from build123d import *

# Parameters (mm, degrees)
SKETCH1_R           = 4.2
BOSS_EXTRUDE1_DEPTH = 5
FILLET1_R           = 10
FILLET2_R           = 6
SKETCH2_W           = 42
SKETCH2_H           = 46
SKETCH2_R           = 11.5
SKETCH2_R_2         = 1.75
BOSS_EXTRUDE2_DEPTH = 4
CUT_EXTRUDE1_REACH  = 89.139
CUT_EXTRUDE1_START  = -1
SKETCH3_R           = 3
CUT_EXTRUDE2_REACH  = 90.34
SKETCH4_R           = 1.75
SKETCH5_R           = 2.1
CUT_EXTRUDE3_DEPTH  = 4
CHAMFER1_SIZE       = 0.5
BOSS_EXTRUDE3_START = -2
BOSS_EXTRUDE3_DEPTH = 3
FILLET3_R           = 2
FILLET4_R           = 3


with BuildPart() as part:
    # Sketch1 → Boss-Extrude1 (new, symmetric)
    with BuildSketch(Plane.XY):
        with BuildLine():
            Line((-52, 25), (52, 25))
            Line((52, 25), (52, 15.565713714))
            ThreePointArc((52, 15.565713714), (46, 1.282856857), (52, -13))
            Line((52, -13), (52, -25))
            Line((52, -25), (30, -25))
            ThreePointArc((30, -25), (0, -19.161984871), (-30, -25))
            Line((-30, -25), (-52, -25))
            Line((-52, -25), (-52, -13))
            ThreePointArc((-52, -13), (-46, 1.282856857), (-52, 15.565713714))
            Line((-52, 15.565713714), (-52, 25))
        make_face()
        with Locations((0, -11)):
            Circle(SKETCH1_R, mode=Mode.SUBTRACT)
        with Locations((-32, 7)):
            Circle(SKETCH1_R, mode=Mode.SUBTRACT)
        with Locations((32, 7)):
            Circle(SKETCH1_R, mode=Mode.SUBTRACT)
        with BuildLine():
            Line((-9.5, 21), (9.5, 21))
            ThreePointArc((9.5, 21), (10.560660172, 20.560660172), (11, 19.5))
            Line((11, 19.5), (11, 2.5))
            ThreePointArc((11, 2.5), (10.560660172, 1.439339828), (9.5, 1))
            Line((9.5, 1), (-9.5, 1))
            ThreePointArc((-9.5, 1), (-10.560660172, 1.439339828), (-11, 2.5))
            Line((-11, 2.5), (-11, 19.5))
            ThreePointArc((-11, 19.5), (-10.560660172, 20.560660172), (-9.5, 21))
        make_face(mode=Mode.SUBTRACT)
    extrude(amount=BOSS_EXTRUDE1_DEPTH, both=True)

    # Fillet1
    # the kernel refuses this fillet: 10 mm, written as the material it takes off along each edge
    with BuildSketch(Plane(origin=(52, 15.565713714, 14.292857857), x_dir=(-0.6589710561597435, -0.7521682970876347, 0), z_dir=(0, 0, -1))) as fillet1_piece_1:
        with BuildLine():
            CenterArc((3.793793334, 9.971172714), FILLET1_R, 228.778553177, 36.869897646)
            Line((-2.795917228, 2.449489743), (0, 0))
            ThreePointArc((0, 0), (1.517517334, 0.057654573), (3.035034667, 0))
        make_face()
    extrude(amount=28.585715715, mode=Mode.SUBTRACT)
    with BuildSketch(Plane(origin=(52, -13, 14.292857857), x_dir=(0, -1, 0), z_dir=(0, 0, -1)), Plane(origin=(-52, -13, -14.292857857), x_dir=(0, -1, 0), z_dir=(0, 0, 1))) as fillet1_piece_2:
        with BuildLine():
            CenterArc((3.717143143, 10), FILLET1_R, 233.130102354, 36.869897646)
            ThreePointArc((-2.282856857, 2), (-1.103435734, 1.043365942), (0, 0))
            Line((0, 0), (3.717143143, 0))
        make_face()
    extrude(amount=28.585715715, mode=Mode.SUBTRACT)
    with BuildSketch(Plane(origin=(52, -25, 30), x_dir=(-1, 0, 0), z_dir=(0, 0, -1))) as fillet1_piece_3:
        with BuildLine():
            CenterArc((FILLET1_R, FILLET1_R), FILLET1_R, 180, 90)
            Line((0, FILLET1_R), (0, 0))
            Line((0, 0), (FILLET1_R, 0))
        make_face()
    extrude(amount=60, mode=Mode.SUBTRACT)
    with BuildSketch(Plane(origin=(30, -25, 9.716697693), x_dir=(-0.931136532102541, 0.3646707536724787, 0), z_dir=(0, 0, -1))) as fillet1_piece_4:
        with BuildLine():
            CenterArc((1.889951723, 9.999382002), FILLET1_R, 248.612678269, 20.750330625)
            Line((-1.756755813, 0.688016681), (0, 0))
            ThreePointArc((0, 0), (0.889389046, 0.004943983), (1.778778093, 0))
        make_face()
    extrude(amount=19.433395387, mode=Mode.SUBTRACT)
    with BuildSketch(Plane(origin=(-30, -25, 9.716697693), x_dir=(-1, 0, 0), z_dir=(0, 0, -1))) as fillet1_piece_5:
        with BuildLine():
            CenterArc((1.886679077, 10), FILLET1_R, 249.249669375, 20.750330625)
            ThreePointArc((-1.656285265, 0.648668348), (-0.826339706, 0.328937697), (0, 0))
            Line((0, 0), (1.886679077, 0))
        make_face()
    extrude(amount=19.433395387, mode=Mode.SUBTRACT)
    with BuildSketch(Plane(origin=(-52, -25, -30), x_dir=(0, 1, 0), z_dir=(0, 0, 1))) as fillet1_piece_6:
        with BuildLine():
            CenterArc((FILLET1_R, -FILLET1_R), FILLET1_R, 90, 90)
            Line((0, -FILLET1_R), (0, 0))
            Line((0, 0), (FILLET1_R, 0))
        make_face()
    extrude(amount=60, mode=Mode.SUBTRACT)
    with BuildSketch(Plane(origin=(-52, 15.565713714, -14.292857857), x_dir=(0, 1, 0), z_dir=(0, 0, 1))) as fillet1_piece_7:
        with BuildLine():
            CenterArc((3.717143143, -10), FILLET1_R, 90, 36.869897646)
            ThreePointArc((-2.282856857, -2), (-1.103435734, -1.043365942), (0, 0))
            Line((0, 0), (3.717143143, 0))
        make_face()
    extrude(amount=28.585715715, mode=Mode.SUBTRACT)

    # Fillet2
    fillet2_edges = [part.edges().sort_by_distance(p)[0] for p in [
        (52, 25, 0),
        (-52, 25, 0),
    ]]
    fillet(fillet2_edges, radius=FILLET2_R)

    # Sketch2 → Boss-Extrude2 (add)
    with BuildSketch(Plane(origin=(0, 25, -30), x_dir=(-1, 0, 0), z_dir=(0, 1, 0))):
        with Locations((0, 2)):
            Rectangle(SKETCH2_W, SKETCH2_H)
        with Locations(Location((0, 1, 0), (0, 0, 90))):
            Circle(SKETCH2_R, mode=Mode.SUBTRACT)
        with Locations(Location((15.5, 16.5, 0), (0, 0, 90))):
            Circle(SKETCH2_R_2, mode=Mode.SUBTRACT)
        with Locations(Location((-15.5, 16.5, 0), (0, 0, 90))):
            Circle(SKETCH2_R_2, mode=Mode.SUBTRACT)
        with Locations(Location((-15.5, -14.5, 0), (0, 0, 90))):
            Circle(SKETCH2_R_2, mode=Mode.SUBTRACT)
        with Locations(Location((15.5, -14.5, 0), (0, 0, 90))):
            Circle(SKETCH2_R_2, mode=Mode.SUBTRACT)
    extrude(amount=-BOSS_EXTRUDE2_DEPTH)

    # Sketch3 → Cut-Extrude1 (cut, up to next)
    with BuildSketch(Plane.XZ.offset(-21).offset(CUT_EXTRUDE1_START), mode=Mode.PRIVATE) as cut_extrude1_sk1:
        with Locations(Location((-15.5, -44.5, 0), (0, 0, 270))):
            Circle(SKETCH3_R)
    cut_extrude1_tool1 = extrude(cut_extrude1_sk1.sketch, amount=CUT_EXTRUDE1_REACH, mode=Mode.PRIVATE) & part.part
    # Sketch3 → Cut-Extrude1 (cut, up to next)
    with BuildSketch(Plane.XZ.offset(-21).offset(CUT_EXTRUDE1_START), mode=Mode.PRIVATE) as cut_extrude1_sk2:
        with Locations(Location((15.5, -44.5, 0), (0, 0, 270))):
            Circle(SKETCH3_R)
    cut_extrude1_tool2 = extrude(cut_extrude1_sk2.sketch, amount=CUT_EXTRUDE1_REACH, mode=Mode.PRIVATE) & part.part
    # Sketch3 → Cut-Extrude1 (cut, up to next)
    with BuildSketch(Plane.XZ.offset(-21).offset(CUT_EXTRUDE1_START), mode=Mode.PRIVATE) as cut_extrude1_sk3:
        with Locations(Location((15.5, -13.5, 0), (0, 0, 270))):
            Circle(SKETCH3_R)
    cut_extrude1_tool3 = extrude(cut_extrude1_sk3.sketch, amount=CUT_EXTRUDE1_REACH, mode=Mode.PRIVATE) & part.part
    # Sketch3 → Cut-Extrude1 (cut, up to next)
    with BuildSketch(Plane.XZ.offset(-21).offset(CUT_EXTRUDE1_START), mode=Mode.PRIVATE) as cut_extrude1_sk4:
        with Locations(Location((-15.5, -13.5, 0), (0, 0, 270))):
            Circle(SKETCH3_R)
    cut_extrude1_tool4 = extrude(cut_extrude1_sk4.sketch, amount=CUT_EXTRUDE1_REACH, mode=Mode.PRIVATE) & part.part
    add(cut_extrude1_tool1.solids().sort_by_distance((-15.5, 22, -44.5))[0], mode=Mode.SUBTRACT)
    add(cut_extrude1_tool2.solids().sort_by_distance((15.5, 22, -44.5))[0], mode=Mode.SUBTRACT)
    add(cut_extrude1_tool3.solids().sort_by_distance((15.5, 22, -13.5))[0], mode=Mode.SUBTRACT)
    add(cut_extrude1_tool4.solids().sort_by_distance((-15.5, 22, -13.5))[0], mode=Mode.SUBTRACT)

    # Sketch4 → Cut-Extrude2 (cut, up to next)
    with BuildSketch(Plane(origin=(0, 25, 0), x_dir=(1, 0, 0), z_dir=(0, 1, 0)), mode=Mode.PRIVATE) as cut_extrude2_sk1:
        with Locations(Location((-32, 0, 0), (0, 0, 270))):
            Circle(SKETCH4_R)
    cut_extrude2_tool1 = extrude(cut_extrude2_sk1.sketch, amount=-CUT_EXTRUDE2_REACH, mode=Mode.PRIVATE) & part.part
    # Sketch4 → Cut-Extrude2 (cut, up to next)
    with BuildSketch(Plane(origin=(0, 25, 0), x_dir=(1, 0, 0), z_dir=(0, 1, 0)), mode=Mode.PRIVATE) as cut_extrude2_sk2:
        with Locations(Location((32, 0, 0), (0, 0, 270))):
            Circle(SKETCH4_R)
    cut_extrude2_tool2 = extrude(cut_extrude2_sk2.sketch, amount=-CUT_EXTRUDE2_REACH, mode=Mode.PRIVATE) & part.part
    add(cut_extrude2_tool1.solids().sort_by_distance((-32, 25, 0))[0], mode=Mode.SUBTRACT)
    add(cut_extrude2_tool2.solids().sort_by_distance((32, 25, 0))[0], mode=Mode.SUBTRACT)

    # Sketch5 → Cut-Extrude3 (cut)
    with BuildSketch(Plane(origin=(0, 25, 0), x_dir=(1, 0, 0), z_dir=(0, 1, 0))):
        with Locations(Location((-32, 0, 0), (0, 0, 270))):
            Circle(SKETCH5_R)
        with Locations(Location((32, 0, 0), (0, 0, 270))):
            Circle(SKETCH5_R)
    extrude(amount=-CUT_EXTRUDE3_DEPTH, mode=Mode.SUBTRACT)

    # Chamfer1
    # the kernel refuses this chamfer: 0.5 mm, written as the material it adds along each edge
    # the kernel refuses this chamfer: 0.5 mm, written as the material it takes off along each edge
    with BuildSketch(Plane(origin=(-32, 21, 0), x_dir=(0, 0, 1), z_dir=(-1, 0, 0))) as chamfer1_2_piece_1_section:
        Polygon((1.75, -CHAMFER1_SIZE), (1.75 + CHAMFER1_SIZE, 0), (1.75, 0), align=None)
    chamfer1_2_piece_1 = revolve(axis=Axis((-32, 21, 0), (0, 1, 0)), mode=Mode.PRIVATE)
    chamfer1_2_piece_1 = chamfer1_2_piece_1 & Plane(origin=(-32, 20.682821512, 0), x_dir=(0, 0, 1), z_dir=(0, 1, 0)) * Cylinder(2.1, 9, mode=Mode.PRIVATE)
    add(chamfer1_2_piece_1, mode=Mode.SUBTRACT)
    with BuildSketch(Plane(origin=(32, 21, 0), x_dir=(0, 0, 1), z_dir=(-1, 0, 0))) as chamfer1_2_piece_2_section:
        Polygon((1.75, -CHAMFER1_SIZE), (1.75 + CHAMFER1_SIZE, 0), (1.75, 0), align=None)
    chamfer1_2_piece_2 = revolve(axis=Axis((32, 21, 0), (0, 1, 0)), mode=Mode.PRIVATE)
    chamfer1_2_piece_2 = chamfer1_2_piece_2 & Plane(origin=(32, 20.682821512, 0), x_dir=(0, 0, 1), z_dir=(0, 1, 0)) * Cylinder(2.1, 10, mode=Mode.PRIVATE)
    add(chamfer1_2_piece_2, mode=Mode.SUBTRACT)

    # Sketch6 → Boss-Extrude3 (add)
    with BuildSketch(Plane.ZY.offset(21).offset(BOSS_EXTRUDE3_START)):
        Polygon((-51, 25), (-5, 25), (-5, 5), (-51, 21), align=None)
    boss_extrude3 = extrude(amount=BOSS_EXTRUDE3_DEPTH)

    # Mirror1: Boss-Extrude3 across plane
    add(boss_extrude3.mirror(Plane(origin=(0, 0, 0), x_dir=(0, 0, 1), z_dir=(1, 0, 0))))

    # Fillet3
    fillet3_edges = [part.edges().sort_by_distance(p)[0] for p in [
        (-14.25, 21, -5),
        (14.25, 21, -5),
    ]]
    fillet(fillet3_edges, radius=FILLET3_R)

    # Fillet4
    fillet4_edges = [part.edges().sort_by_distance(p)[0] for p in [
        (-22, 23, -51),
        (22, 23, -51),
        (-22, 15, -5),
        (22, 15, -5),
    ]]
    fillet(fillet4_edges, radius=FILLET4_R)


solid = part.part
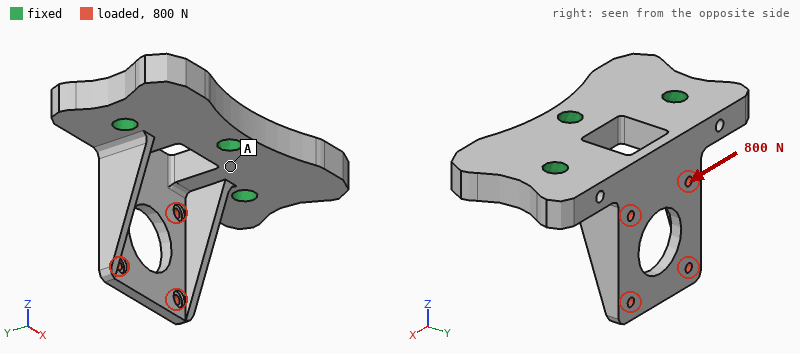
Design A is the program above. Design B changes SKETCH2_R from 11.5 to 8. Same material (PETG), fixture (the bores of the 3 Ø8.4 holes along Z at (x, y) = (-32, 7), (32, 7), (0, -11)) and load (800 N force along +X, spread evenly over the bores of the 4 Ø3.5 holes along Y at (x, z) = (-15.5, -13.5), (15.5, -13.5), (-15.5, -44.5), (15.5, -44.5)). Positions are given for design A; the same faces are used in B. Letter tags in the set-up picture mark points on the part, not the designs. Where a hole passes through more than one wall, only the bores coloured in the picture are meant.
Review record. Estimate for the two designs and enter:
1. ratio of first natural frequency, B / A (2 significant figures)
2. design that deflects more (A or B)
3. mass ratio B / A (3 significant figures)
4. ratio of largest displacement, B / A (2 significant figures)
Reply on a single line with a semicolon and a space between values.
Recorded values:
0.97; A; 1.02; 0.84
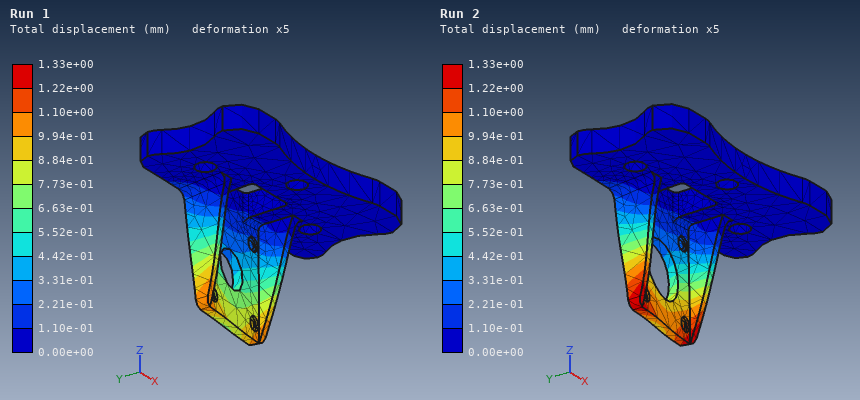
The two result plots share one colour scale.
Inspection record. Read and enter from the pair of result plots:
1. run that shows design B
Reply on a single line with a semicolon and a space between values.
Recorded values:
Run 1
